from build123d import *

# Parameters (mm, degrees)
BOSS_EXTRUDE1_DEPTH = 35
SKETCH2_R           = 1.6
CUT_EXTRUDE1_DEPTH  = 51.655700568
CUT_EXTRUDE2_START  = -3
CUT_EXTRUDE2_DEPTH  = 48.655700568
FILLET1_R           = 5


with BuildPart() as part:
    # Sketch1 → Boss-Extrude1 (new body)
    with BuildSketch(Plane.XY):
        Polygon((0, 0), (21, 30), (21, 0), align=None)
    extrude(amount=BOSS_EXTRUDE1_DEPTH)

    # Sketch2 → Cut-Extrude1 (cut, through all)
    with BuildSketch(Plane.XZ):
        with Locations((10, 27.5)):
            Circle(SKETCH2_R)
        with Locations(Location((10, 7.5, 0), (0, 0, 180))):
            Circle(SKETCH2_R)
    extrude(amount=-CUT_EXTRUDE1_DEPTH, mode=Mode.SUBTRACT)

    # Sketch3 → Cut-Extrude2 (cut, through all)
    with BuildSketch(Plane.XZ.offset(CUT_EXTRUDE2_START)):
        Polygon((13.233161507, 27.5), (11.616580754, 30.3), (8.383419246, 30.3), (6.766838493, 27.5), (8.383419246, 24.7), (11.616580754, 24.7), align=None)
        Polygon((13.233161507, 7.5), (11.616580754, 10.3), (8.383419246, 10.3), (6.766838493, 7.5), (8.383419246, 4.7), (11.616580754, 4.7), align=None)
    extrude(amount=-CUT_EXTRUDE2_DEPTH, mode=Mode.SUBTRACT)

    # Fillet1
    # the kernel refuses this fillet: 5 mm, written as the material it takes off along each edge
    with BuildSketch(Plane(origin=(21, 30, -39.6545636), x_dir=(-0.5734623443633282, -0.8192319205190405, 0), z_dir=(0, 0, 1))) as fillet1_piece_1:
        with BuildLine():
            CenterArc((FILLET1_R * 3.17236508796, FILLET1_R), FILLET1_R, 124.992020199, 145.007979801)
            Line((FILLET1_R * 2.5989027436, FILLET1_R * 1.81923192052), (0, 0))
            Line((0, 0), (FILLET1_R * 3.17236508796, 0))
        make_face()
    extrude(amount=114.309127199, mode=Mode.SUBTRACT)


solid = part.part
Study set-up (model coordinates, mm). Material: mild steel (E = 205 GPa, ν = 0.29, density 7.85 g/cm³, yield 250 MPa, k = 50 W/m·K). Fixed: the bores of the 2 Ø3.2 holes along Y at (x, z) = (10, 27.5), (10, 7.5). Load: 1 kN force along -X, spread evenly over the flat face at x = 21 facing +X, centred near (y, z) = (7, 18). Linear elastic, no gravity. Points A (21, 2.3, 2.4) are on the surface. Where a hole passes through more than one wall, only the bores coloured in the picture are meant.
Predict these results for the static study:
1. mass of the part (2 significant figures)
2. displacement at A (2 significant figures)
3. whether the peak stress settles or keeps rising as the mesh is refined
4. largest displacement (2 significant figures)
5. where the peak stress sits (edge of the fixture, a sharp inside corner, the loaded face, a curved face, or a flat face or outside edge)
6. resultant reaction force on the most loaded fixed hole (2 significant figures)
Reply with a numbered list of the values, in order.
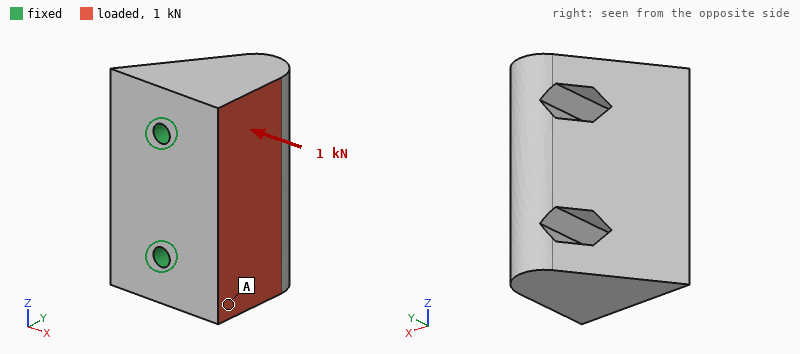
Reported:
1. 68 g
2. 5.5 µm
3. keeps rising
4. 9.9 µm
5. edge of the fixture
6. 500 N
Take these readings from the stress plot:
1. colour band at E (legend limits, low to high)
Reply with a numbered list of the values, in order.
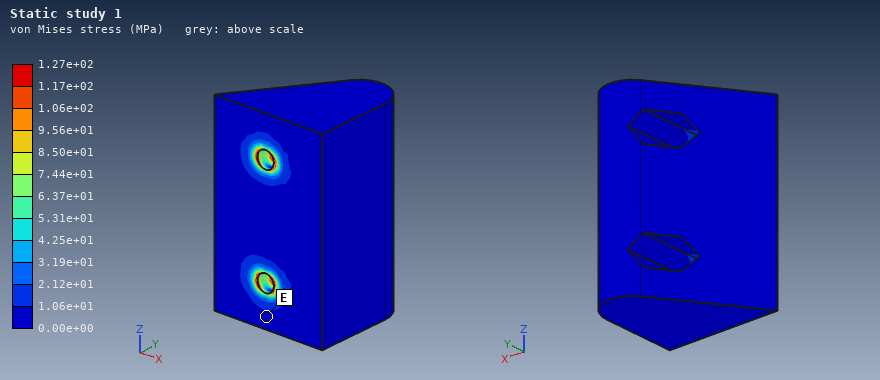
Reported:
1. 0.00e+00 to 1.06e+01 MPa
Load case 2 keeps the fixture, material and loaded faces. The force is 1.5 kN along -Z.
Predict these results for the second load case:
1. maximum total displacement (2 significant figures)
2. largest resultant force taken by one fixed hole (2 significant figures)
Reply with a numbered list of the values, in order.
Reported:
1. 3.1 µm
2. 1.1 kN
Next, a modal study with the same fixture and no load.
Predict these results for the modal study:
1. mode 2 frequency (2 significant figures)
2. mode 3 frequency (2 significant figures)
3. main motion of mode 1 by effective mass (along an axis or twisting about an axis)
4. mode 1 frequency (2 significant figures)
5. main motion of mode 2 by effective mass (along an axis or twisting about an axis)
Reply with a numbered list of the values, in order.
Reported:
1. 18 kHz
2. 21 kHz
3. along X
4. 6300 Hz
5. along Z
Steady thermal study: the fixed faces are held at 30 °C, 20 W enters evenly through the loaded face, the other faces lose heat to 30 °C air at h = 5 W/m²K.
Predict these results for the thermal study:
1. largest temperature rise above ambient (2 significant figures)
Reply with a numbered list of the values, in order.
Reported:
1. 22 K
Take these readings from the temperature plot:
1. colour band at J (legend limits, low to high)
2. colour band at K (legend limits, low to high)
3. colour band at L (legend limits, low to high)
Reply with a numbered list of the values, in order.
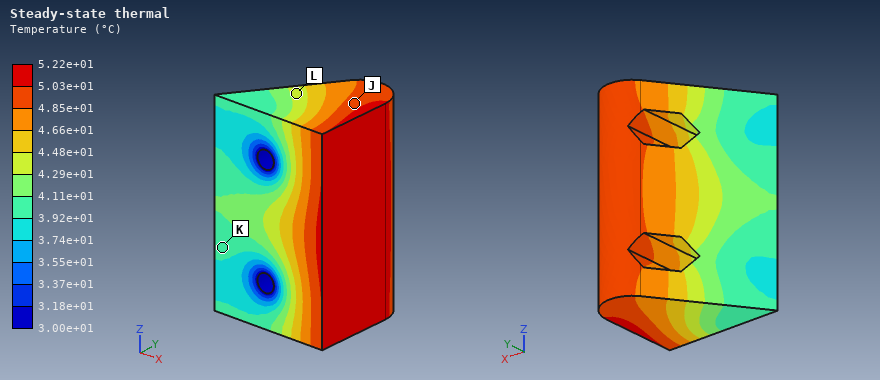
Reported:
1. 4.85e+01 to 5.03e+01 °C
2. 3.92e+01 to 4.11e+01 °C
3. 4.29e+01 to 4.48e+01 °C
